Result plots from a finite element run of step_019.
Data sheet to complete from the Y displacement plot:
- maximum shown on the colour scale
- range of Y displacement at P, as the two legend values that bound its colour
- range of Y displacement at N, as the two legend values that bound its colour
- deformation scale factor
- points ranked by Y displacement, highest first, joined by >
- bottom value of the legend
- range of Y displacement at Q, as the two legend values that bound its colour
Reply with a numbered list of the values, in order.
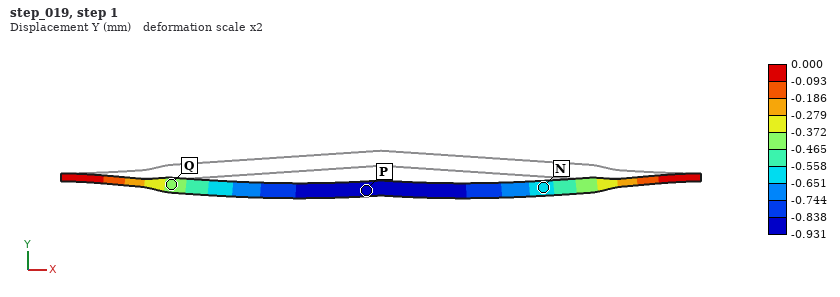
1. 0.000 mm
2. -0.931 to -0.838 mm
3. -0.651 to -0.558 mm
4. 2
5. Q > N > P
6. -0.931 mm
7. -0.465 to -0.372 mm
